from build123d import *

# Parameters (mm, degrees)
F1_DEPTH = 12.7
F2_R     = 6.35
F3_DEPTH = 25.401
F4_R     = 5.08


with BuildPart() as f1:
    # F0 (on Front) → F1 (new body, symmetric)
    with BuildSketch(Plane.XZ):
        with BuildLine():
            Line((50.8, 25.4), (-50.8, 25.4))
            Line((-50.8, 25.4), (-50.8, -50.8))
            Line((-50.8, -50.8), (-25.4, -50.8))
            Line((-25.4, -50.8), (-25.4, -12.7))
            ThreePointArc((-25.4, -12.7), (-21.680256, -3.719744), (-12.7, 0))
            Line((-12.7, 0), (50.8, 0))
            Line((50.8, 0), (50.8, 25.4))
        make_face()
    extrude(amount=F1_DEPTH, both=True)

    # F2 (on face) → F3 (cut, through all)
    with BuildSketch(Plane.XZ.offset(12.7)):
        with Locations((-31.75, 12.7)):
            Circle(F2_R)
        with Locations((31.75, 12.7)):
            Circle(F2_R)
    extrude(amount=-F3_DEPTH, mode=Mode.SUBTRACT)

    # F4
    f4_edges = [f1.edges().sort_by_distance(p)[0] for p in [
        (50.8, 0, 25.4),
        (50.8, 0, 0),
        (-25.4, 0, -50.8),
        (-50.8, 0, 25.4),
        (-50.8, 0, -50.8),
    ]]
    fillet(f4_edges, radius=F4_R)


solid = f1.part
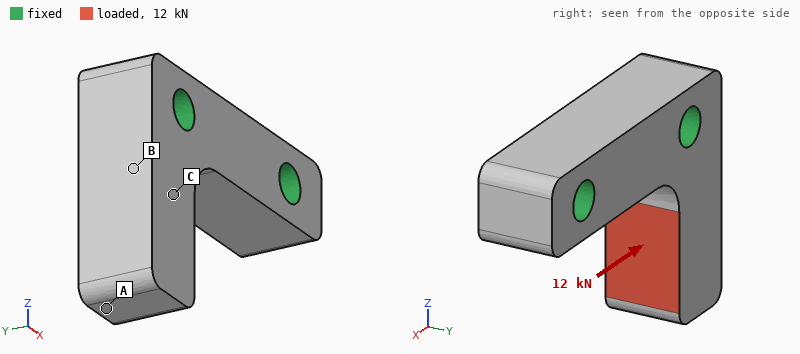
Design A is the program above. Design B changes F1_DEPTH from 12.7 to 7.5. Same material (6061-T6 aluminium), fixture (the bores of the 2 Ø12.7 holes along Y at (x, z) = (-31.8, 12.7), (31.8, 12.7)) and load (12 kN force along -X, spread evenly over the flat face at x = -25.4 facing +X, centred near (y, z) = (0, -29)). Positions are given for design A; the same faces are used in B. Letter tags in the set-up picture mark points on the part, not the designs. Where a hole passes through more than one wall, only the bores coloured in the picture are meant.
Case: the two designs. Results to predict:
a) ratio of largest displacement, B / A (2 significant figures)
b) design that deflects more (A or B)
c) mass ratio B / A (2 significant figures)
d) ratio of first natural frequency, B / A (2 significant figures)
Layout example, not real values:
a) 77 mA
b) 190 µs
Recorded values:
a) 1.7
b) B
c) 0.59
d) 0.66
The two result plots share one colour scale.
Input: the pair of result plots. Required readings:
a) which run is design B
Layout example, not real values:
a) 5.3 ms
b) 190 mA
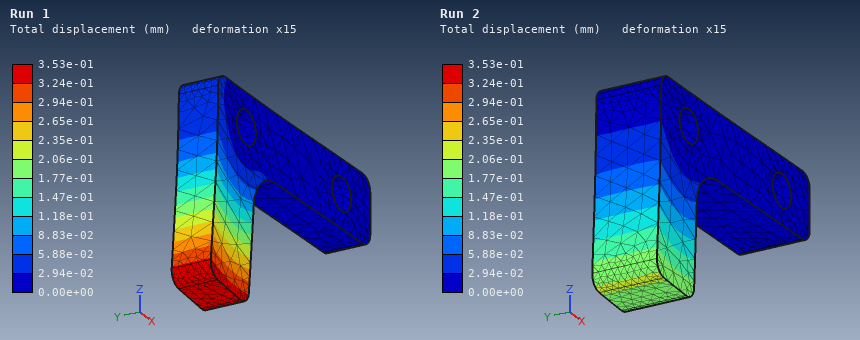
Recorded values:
a) Run 1
